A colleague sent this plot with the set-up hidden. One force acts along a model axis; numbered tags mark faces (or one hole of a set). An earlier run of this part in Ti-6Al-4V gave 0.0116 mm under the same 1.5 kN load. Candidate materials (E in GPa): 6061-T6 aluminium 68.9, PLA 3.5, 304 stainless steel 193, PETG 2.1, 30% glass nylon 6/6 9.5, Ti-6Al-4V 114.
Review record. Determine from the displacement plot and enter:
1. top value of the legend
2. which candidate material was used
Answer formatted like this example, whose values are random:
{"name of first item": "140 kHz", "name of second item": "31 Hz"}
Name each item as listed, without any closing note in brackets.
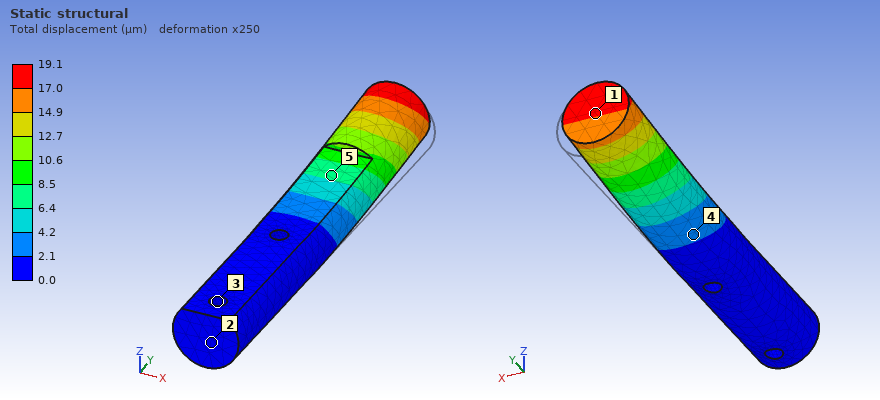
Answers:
{"top value of the legend": "19.1 µm", "which candidate material was used": "6061-T6 aluminium"}
